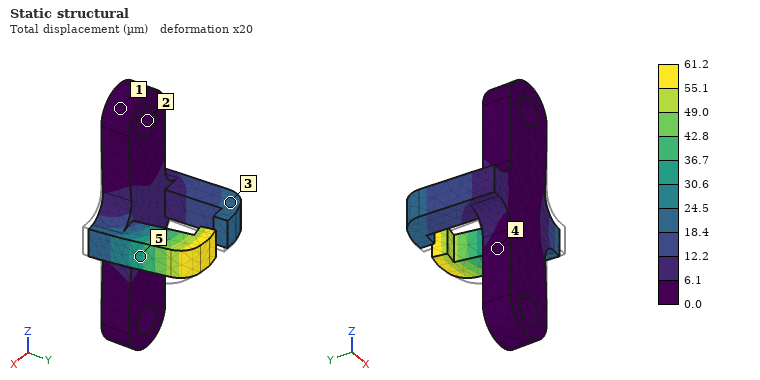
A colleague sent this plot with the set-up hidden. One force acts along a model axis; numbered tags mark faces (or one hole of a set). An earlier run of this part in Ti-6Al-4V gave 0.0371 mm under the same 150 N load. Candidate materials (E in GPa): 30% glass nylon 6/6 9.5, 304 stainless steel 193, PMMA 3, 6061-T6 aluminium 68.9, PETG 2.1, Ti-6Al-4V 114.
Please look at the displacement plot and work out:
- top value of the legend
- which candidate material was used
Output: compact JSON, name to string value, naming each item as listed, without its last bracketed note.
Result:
{"top value of the legend": "61.2 µm", "which candidate material was used": "6061-T6 aluminium"}
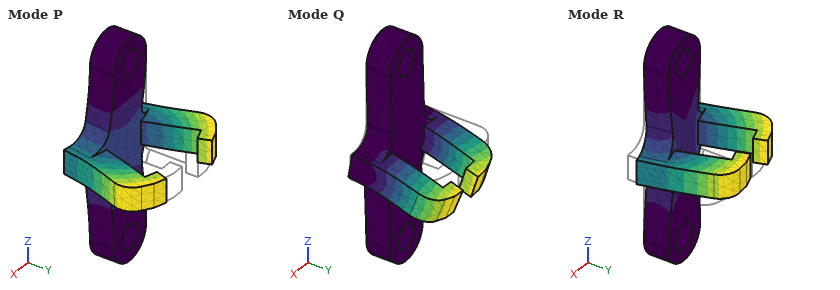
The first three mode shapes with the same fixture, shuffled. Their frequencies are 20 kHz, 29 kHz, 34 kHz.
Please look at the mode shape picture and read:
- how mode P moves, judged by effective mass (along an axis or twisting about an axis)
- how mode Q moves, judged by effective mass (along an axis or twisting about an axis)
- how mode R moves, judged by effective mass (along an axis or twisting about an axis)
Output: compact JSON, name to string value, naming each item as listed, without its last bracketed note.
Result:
{"how mode P moves, judged by effective mass": "along Y", "how mode Q moves, judged by effective mass": "along Z", "how mode R moves, judged by effective mass": "along X"}
